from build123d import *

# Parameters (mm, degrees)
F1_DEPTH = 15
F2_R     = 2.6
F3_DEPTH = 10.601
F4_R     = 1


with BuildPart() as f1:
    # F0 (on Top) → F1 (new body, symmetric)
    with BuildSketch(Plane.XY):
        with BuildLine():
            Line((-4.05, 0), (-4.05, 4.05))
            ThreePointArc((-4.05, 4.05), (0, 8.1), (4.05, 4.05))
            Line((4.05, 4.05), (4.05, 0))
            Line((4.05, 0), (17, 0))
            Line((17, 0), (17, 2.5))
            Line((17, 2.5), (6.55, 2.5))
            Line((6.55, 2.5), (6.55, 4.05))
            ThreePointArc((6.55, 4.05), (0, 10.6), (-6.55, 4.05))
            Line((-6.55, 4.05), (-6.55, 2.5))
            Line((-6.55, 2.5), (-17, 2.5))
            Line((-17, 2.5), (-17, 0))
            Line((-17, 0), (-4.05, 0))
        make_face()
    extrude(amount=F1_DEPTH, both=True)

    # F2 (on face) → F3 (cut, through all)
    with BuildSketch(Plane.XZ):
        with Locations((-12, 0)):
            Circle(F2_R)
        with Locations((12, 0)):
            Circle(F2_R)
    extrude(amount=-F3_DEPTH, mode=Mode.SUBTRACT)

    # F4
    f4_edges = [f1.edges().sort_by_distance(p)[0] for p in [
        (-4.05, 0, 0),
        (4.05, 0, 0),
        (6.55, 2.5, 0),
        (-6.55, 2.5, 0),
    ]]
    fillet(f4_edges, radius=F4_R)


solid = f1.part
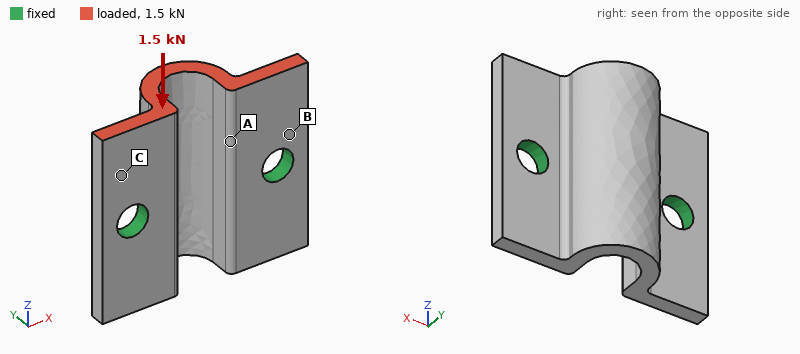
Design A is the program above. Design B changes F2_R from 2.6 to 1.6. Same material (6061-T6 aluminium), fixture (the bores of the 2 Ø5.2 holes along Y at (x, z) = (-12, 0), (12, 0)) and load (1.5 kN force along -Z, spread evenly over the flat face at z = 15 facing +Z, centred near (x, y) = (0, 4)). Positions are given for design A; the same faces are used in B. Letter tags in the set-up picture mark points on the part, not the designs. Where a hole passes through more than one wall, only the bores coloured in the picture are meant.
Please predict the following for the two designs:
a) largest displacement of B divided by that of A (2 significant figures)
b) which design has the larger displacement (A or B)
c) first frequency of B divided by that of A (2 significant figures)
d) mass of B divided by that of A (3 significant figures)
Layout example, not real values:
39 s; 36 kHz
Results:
1.7; B; 0.76; 1.02
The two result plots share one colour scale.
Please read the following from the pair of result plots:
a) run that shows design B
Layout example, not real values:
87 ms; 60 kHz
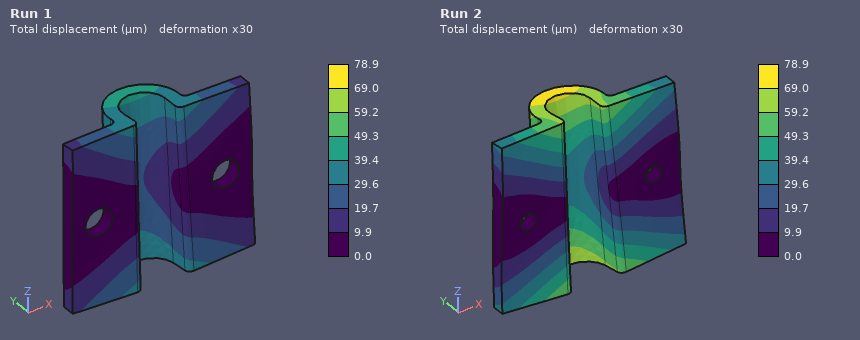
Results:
Run 2
